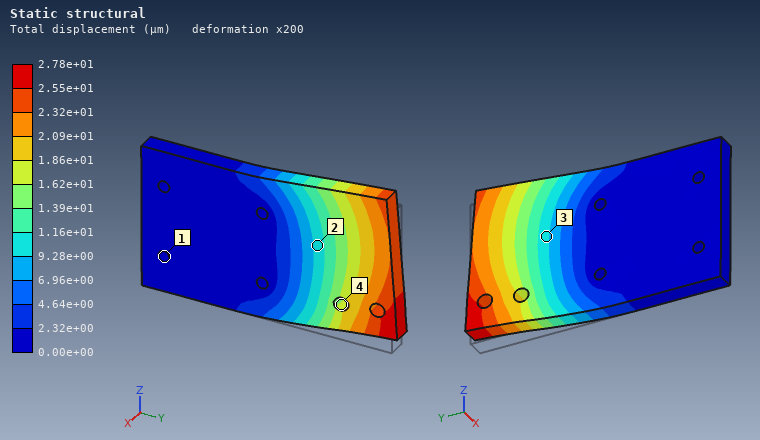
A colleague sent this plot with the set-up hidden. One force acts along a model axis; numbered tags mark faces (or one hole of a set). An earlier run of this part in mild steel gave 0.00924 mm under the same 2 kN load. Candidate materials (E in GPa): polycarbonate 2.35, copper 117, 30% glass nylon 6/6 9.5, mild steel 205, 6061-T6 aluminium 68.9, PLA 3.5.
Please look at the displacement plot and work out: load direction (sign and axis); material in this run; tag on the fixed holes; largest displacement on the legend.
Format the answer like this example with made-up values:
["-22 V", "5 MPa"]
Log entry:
["+Z", "6061-T6 aluminium", "1", "2.78e+01 µm"]
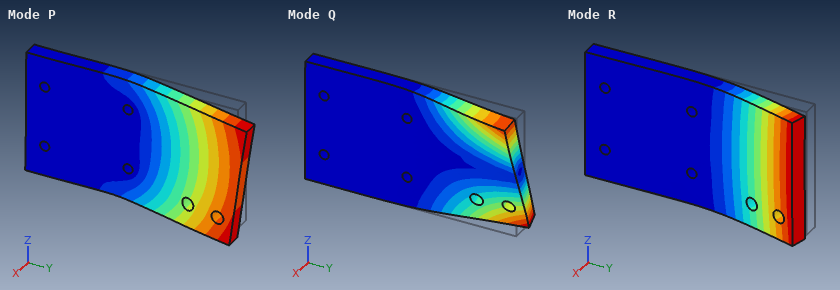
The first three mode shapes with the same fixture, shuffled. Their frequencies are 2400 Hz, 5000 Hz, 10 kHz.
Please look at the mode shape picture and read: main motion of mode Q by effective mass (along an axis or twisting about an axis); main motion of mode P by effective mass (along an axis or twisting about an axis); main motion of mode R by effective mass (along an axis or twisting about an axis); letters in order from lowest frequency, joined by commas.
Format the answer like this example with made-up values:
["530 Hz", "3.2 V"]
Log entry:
["twisting about Y", "along Z", "along X", "R, Q, P"]
